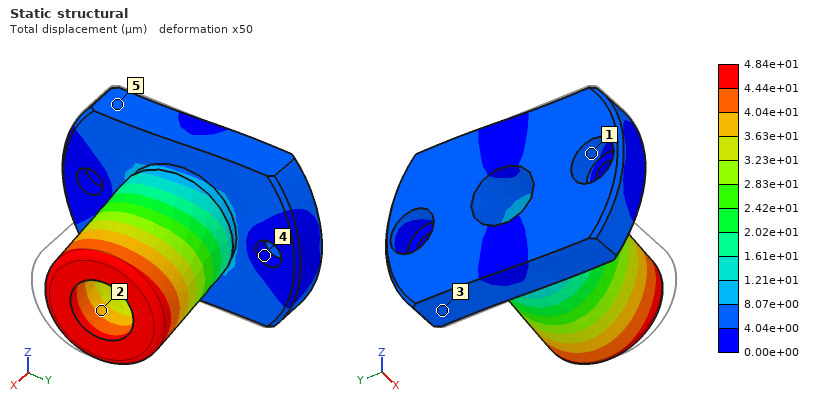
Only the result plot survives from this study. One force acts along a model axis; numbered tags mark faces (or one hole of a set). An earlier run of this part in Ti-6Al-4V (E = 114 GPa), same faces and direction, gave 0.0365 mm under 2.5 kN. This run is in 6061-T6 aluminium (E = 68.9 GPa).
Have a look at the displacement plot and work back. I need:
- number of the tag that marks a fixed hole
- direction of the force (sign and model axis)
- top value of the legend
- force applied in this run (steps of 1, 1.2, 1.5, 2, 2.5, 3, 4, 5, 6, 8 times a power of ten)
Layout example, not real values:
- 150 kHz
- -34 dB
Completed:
- 4
- +Y
- 4.84e+01 µm
- 2 kN
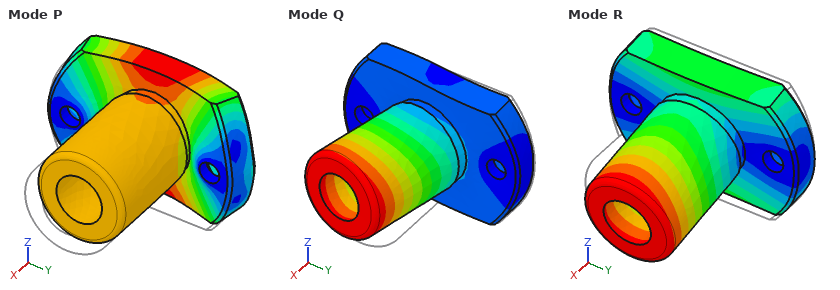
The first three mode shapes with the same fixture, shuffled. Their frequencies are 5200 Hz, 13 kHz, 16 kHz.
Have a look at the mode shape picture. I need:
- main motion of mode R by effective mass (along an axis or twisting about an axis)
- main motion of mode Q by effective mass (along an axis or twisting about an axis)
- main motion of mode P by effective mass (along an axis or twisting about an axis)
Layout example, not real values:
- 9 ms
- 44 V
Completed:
- along Z
- along Y
- along X
